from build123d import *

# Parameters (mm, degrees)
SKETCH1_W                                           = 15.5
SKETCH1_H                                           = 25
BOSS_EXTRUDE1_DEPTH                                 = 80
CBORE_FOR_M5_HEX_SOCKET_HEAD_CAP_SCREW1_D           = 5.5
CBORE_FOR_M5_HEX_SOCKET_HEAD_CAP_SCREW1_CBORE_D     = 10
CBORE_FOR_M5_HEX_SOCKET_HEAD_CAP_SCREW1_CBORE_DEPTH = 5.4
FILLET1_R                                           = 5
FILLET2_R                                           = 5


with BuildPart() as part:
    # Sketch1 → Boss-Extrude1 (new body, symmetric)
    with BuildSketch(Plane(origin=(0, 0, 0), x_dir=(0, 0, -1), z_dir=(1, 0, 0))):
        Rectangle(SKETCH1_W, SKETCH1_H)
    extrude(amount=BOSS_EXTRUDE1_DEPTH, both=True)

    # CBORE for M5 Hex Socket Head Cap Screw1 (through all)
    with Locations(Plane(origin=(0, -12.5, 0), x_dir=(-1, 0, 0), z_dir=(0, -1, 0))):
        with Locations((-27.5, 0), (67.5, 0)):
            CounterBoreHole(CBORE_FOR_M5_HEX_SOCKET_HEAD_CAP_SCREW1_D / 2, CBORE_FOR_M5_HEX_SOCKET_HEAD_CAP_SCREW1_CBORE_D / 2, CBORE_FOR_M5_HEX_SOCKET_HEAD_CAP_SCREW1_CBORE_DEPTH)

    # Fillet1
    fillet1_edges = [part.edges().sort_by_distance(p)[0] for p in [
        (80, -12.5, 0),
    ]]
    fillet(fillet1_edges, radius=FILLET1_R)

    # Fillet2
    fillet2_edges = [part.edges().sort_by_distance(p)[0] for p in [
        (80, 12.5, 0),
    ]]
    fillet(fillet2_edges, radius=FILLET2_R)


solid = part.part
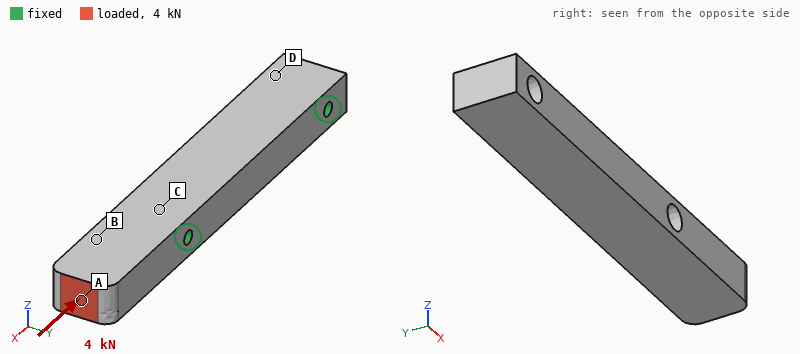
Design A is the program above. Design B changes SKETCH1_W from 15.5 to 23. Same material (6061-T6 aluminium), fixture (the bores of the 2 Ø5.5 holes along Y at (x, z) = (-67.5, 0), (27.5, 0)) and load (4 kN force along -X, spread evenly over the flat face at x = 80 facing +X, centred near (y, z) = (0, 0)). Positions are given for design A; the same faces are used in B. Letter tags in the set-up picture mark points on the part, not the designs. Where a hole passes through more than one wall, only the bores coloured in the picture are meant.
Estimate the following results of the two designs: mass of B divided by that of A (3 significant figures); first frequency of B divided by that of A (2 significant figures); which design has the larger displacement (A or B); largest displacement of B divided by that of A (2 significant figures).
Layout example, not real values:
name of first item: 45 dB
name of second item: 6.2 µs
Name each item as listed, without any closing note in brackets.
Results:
mass of B divided by that of A: 1.50
first frequency of B divided by that of A: 1.2
which design has the larger displacement: A
largest displacement of B divided by that of A: 0.71
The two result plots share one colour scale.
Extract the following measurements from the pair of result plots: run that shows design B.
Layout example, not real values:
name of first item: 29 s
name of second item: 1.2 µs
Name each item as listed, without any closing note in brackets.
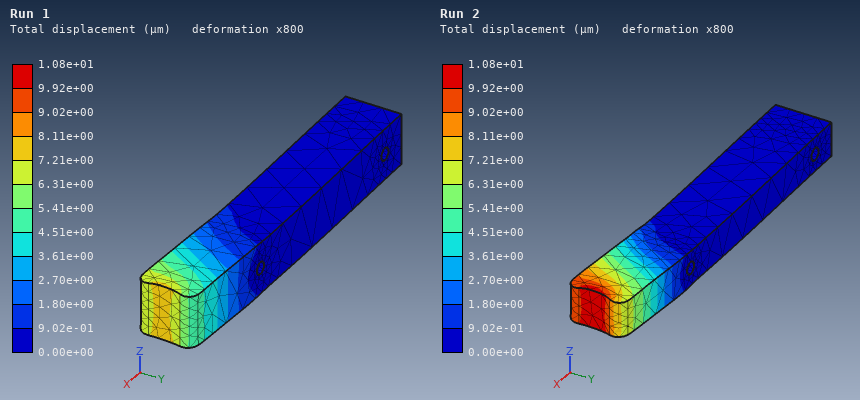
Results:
run that shows design B: Run 1
